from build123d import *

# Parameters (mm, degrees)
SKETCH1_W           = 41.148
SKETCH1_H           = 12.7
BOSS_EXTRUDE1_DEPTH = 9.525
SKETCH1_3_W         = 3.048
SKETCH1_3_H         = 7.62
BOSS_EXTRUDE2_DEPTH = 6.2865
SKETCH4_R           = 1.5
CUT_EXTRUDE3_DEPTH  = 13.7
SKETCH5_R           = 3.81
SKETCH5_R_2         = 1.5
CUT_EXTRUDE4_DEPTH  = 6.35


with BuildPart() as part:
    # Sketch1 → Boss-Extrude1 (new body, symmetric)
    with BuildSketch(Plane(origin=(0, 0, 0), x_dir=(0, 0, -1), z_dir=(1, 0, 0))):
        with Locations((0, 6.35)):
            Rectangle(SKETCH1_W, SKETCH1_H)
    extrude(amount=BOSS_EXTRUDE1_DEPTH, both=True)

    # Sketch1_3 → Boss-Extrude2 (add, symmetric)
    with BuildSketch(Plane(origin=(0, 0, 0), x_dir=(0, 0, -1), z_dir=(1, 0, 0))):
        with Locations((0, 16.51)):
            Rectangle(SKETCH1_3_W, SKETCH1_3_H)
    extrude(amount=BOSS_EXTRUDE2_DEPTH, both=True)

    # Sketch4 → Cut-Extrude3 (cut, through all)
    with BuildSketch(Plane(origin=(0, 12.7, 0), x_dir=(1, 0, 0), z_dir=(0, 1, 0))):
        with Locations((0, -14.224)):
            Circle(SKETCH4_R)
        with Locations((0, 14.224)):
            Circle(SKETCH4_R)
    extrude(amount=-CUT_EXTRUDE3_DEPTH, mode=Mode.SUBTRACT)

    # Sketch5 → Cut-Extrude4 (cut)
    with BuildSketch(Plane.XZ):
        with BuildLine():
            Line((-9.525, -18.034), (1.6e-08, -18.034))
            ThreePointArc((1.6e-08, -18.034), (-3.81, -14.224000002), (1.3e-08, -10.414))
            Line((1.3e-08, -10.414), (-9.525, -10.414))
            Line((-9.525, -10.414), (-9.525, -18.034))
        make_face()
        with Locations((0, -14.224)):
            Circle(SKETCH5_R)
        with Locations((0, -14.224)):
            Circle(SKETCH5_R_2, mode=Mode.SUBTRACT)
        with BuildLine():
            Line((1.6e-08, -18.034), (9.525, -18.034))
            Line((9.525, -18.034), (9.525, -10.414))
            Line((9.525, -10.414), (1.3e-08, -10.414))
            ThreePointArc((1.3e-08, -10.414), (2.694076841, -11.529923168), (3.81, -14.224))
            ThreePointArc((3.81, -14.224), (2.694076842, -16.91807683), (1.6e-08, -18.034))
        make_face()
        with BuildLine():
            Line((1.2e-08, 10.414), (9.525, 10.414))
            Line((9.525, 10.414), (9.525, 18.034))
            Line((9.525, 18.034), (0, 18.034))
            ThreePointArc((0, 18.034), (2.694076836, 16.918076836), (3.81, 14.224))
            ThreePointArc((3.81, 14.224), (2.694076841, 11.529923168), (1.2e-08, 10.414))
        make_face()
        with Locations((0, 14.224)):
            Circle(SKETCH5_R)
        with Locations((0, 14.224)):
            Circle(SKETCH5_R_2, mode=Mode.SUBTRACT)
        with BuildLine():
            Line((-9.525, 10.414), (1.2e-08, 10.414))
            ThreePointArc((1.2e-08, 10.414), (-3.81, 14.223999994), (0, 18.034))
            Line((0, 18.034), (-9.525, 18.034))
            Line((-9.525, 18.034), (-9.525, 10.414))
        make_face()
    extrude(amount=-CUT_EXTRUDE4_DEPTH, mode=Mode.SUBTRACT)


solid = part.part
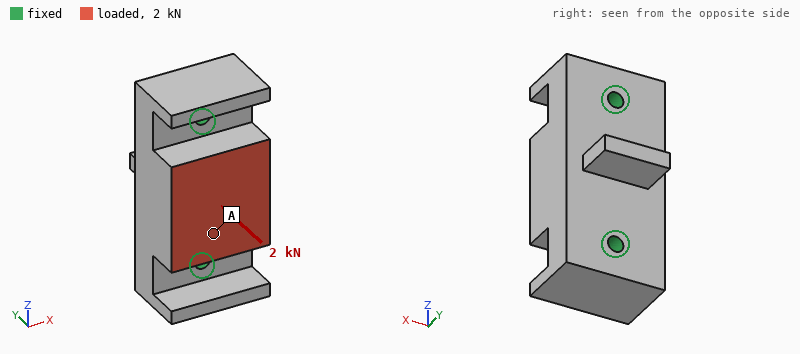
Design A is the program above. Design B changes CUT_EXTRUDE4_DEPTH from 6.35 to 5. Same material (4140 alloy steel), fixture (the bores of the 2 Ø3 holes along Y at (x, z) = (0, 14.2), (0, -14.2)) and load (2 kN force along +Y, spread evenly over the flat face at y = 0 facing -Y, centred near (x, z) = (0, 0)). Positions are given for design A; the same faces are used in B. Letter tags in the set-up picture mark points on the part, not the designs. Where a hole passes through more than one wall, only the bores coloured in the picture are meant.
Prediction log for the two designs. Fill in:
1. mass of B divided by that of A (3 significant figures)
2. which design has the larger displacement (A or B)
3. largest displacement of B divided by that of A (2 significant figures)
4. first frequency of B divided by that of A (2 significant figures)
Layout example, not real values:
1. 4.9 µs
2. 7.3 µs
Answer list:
1. 1.04
2. A
3. 0.84
4. 1.3
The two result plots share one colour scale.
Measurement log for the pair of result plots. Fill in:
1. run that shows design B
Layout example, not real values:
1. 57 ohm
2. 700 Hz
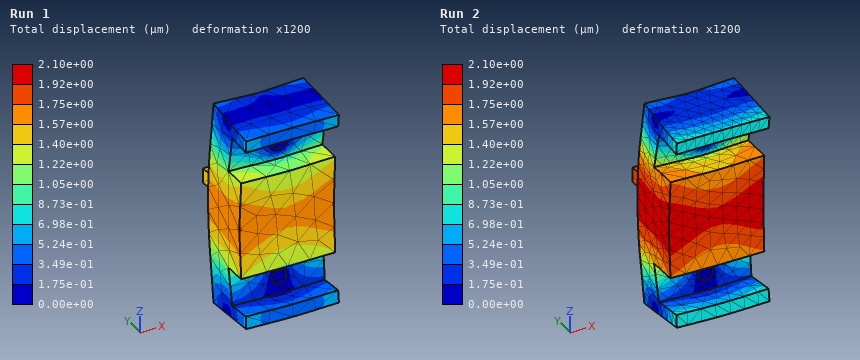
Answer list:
1. Run 1
